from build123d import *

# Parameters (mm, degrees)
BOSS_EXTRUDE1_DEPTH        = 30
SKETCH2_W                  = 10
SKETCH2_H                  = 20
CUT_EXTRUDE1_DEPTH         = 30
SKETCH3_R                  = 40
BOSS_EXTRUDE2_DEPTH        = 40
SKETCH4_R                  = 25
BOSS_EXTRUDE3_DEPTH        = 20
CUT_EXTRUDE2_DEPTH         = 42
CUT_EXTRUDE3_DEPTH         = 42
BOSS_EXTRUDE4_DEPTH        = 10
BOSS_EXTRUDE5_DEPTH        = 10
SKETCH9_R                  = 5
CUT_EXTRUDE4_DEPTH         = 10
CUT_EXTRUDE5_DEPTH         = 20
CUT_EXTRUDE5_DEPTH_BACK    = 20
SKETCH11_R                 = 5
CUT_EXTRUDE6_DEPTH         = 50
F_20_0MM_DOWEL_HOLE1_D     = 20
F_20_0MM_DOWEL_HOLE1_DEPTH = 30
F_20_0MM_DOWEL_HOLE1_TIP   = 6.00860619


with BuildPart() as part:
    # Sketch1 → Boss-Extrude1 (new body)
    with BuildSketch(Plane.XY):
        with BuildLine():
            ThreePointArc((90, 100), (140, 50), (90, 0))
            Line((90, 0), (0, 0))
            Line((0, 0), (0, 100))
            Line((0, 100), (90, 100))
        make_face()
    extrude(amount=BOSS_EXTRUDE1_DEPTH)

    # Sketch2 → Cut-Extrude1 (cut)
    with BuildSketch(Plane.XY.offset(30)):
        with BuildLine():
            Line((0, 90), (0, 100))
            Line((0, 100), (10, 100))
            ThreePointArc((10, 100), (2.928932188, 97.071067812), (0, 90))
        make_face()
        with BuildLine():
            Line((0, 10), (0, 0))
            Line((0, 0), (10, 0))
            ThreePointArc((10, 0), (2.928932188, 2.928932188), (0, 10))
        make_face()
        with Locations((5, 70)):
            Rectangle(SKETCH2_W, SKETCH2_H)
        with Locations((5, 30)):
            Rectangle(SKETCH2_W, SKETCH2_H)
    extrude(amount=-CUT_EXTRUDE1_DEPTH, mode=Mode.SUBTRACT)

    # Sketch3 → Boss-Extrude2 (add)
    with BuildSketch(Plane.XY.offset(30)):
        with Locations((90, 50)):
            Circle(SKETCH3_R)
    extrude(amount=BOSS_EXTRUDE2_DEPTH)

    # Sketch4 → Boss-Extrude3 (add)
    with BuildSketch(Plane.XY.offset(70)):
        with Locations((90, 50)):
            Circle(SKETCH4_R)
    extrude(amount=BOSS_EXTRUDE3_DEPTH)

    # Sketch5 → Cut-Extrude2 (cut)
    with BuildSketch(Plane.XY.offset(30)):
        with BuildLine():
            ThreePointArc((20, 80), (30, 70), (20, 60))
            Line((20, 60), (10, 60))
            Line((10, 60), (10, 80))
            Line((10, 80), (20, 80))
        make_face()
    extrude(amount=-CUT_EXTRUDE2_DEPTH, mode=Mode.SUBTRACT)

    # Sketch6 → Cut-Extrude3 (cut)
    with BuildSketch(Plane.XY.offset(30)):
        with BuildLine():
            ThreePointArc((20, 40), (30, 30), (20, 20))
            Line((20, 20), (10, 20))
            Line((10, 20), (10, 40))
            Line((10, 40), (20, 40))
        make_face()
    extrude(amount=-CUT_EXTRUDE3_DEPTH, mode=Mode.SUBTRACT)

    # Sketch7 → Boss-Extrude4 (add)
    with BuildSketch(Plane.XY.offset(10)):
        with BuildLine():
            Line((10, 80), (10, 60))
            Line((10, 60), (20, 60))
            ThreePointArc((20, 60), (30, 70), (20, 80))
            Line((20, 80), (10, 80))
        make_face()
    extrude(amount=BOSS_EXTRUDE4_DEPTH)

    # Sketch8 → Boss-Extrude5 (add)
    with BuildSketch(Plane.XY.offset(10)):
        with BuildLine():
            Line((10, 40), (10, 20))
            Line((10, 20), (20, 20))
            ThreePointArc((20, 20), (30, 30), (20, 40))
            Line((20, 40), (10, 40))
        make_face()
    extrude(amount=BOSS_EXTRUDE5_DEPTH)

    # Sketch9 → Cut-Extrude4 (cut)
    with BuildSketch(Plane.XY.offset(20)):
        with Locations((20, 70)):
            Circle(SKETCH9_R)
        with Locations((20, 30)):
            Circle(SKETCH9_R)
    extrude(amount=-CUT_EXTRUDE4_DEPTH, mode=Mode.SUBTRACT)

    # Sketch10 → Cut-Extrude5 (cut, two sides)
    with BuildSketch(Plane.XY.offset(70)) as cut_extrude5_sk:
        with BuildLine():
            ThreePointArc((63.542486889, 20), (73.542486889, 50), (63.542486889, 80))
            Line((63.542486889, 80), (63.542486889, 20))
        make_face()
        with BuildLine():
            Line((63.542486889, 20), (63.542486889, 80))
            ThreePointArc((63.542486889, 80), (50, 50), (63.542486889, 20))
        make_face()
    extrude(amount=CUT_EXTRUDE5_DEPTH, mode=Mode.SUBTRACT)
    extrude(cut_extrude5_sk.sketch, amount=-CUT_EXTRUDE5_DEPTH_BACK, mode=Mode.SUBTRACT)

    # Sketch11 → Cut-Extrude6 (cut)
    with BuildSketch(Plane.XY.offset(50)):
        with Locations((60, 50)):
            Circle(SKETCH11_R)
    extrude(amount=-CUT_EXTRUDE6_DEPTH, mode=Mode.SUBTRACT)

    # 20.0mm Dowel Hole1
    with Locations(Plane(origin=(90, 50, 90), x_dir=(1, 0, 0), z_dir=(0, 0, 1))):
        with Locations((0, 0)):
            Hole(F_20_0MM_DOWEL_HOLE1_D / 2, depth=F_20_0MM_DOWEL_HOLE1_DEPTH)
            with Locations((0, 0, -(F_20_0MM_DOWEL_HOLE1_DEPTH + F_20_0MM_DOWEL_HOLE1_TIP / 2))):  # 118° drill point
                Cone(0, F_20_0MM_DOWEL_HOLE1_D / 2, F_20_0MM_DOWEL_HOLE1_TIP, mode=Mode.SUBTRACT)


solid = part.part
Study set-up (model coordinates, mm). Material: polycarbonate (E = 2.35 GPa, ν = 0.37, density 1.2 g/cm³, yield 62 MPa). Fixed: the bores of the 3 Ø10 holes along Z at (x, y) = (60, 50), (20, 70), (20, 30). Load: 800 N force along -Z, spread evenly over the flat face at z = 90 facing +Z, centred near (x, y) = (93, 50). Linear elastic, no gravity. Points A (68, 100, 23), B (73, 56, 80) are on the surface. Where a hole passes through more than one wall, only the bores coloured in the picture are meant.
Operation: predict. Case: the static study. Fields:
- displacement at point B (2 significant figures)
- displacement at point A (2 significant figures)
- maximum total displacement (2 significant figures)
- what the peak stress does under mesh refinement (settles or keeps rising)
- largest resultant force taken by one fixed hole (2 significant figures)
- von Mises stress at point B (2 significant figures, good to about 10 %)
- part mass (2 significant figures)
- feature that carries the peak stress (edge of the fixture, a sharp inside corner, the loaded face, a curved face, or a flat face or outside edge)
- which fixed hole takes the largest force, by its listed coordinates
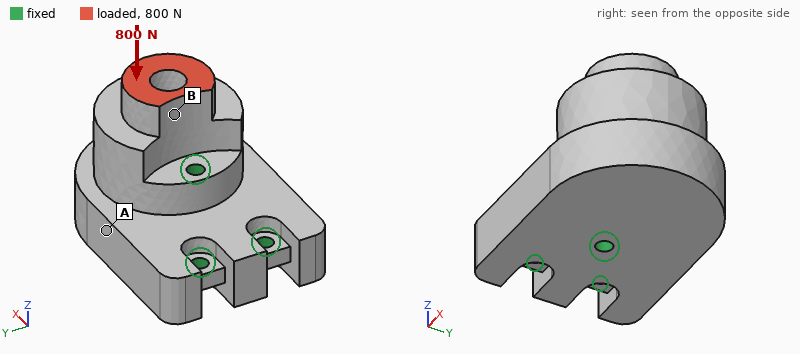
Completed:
33 µm
10 µm
56 µm
keeps rising
890 N
0.51 MPa
670 g
edge of the fixture
(60, 50)
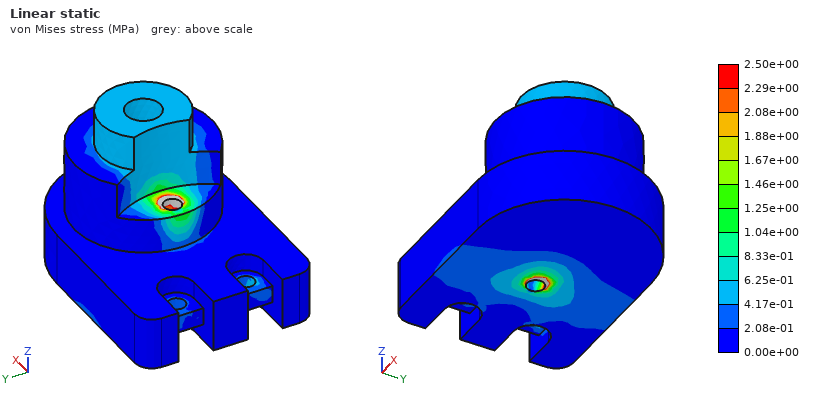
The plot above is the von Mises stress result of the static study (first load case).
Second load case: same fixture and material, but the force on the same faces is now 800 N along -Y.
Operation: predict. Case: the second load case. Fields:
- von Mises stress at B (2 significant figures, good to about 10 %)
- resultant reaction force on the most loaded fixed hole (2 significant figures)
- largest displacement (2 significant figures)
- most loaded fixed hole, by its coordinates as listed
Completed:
2.0 MPa
1.1 kN
0.15 mm
(60, 50)
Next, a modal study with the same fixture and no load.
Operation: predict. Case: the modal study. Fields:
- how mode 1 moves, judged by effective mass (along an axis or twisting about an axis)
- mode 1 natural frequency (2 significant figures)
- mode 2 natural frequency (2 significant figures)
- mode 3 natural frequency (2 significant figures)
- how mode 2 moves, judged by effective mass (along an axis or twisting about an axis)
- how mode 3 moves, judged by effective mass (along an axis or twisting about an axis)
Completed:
along Z
1000 Hz
1100 Hz
1400 Hz
along Y
twisting about X
